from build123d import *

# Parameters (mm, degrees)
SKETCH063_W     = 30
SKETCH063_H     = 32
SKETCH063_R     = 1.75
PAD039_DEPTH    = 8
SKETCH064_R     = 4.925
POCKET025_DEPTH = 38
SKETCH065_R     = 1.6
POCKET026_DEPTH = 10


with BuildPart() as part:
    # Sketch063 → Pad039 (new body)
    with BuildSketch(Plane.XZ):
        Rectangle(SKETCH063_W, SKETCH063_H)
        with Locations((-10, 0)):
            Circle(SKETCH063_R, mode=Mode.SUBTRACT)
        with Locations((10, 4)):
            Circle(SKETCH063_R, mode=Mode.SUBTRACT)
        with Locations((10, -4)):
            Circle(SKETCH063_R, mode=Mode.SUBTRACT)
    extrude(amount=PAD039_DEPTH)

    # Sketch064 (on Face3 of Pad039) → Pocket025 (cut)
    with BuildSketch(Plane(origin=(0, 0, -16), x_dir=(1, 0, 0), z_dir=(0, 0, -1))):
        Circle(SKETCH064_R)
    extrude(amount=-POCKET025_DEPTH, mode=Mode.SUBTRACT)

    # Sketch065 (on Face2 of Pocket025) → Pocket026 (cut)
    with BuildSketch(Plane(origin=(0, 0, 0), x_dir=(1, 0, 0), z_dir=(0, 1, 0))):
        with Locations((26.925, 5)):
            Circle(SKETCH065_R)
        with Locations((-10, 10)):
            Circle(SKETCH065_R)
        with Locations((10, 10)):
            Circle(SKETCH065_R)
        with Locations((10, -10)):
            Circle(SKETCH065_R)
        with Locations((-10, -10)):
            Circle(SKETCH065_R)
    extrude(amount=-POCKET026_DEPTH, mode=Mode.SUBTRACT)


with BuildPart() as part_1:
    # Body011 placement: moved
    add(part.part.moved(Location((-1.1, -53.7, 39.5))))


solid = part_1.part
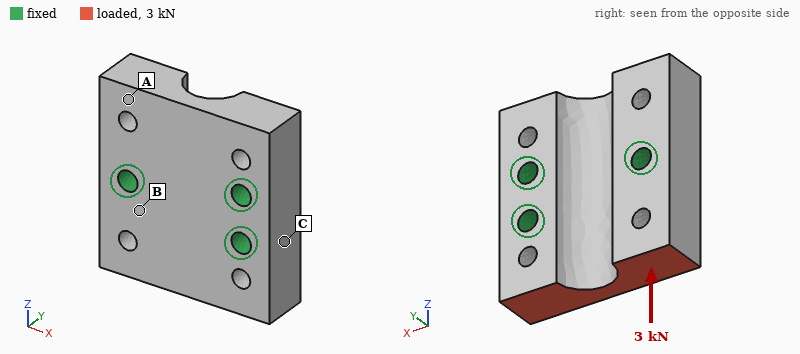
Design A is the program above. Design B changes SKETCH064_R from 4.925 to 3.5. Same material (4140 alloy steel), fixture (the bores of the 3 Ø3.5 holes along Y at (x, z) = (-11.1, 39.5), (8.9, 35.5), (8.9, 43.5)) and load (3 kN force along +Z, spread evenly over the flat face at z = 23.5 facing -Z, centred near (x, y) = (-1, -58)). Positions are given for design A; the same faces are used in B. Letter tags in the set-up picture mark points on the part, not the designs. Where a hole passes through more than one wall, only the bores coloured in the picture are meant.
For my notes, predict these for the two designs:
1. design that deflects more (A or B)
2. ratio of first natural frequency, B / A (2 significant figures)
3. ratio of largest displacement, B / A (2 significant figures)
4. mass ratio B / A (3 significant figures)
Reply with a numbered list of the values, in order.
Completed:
1. A
2. 1.00
3. 0.92
4. 1.10
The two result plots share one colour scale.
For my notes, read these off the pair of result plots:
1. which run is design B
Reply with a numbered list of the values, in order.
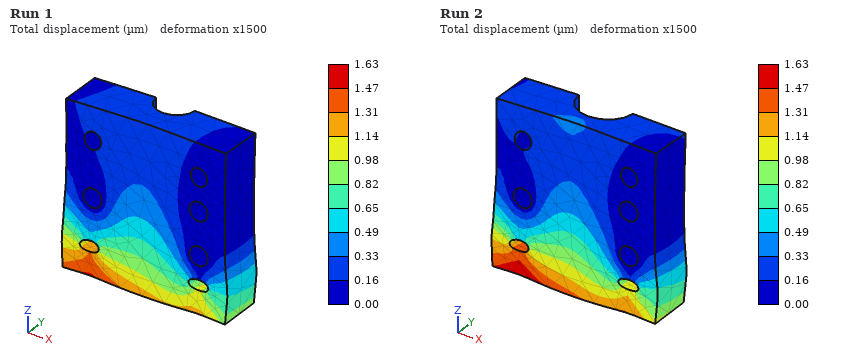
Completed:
1. Run 1
